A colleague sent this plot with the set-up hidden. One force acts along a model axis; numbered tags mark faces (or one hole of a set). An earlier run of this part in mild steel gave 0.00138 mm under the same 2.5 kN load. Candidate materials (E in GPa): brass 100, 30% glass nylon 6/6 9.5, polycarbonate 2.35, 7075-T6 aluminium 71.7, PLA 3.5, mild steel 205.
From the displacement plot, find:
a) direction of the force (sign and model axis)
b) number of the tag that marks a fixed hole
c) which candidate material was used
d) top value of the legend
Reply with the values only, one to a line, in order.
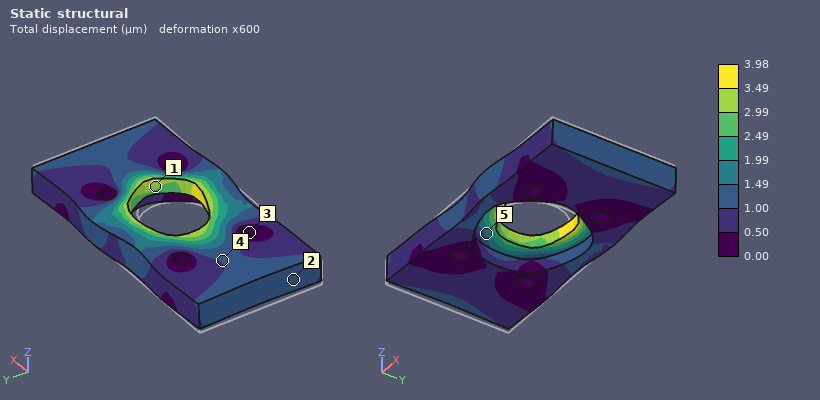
+X
3
7075-T6 aluminium
3.98 µm
